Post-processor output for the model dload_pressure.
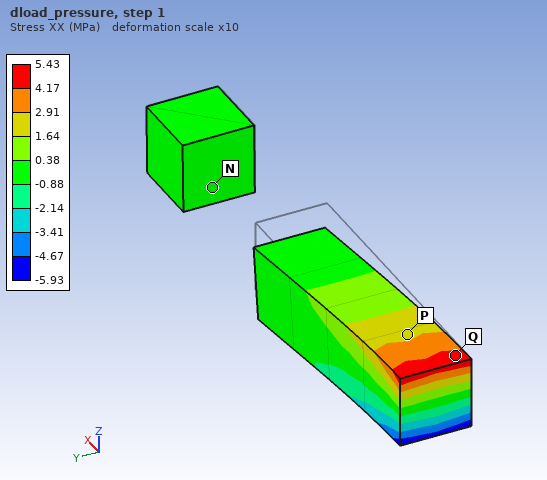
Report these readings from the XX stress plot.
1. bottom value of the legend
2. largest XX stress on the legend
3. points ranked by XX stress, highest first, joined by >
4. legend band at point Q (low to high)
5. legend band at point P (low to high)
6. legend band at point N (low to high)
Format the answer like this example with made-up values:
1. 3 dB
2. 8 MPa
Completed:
1. -5.93 MPa
2. 5.43 MPa
3. Q > P > N
4. 4.17 to 5.43 MPa
5. 1.64 to 2.91 MPa
6. -0.88 to 0.38 MPa
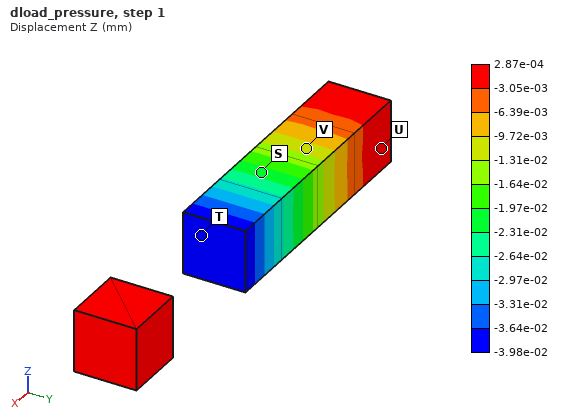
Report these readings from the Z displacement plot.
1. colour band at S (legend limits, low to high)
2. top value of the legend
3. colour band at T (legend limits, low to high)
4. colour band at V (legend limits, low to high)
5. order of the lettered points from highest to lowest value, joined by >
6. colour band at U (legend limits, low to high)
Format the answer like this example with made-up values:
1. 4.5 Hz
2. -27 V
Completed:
1. -2.31e-02 to -1.97e-02 mm
2. 2.87e-04 mm
3. -3.98e-02 to -3.64e-02 mm
4. -1.31e-02 to -9.72e-03 mm
5. U > V > S > T
6. -3.05e-03 to 2.87e-04 mm
